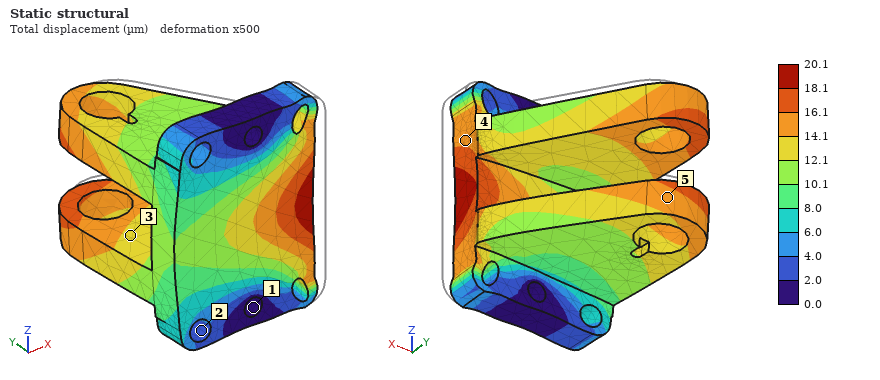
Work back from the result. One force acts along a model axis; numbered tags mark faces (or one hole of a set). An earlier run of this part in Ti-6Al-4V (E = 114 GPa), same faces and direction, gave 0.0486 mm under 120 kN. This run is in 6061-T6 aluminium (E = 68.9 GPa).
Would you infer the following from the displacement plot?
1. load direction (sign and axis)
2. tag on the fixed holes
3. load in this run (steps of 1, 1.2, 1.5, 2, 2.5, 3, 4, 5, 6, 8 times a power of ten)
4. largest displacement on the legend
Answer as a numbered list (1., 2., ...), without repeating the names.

1. -X
2. 1
3. 30 kN
4. 20.1 µm
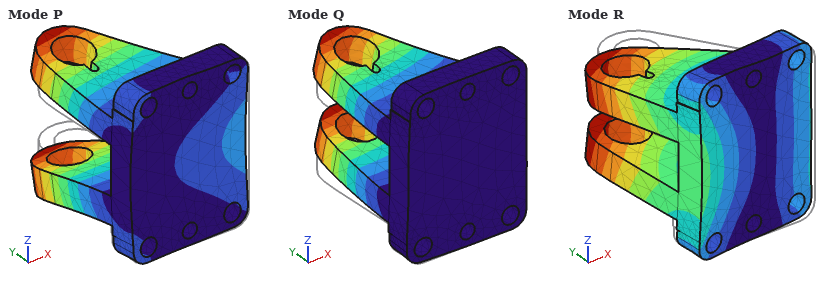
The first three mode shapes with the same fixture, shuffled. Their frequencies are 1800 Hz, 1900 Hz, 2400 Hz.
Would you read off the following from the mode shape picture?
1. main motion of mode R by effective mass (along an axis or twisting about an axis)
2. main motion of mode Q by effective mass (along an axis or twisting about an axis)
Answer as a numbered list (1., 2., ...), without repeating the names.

1. along X
2. along Z
